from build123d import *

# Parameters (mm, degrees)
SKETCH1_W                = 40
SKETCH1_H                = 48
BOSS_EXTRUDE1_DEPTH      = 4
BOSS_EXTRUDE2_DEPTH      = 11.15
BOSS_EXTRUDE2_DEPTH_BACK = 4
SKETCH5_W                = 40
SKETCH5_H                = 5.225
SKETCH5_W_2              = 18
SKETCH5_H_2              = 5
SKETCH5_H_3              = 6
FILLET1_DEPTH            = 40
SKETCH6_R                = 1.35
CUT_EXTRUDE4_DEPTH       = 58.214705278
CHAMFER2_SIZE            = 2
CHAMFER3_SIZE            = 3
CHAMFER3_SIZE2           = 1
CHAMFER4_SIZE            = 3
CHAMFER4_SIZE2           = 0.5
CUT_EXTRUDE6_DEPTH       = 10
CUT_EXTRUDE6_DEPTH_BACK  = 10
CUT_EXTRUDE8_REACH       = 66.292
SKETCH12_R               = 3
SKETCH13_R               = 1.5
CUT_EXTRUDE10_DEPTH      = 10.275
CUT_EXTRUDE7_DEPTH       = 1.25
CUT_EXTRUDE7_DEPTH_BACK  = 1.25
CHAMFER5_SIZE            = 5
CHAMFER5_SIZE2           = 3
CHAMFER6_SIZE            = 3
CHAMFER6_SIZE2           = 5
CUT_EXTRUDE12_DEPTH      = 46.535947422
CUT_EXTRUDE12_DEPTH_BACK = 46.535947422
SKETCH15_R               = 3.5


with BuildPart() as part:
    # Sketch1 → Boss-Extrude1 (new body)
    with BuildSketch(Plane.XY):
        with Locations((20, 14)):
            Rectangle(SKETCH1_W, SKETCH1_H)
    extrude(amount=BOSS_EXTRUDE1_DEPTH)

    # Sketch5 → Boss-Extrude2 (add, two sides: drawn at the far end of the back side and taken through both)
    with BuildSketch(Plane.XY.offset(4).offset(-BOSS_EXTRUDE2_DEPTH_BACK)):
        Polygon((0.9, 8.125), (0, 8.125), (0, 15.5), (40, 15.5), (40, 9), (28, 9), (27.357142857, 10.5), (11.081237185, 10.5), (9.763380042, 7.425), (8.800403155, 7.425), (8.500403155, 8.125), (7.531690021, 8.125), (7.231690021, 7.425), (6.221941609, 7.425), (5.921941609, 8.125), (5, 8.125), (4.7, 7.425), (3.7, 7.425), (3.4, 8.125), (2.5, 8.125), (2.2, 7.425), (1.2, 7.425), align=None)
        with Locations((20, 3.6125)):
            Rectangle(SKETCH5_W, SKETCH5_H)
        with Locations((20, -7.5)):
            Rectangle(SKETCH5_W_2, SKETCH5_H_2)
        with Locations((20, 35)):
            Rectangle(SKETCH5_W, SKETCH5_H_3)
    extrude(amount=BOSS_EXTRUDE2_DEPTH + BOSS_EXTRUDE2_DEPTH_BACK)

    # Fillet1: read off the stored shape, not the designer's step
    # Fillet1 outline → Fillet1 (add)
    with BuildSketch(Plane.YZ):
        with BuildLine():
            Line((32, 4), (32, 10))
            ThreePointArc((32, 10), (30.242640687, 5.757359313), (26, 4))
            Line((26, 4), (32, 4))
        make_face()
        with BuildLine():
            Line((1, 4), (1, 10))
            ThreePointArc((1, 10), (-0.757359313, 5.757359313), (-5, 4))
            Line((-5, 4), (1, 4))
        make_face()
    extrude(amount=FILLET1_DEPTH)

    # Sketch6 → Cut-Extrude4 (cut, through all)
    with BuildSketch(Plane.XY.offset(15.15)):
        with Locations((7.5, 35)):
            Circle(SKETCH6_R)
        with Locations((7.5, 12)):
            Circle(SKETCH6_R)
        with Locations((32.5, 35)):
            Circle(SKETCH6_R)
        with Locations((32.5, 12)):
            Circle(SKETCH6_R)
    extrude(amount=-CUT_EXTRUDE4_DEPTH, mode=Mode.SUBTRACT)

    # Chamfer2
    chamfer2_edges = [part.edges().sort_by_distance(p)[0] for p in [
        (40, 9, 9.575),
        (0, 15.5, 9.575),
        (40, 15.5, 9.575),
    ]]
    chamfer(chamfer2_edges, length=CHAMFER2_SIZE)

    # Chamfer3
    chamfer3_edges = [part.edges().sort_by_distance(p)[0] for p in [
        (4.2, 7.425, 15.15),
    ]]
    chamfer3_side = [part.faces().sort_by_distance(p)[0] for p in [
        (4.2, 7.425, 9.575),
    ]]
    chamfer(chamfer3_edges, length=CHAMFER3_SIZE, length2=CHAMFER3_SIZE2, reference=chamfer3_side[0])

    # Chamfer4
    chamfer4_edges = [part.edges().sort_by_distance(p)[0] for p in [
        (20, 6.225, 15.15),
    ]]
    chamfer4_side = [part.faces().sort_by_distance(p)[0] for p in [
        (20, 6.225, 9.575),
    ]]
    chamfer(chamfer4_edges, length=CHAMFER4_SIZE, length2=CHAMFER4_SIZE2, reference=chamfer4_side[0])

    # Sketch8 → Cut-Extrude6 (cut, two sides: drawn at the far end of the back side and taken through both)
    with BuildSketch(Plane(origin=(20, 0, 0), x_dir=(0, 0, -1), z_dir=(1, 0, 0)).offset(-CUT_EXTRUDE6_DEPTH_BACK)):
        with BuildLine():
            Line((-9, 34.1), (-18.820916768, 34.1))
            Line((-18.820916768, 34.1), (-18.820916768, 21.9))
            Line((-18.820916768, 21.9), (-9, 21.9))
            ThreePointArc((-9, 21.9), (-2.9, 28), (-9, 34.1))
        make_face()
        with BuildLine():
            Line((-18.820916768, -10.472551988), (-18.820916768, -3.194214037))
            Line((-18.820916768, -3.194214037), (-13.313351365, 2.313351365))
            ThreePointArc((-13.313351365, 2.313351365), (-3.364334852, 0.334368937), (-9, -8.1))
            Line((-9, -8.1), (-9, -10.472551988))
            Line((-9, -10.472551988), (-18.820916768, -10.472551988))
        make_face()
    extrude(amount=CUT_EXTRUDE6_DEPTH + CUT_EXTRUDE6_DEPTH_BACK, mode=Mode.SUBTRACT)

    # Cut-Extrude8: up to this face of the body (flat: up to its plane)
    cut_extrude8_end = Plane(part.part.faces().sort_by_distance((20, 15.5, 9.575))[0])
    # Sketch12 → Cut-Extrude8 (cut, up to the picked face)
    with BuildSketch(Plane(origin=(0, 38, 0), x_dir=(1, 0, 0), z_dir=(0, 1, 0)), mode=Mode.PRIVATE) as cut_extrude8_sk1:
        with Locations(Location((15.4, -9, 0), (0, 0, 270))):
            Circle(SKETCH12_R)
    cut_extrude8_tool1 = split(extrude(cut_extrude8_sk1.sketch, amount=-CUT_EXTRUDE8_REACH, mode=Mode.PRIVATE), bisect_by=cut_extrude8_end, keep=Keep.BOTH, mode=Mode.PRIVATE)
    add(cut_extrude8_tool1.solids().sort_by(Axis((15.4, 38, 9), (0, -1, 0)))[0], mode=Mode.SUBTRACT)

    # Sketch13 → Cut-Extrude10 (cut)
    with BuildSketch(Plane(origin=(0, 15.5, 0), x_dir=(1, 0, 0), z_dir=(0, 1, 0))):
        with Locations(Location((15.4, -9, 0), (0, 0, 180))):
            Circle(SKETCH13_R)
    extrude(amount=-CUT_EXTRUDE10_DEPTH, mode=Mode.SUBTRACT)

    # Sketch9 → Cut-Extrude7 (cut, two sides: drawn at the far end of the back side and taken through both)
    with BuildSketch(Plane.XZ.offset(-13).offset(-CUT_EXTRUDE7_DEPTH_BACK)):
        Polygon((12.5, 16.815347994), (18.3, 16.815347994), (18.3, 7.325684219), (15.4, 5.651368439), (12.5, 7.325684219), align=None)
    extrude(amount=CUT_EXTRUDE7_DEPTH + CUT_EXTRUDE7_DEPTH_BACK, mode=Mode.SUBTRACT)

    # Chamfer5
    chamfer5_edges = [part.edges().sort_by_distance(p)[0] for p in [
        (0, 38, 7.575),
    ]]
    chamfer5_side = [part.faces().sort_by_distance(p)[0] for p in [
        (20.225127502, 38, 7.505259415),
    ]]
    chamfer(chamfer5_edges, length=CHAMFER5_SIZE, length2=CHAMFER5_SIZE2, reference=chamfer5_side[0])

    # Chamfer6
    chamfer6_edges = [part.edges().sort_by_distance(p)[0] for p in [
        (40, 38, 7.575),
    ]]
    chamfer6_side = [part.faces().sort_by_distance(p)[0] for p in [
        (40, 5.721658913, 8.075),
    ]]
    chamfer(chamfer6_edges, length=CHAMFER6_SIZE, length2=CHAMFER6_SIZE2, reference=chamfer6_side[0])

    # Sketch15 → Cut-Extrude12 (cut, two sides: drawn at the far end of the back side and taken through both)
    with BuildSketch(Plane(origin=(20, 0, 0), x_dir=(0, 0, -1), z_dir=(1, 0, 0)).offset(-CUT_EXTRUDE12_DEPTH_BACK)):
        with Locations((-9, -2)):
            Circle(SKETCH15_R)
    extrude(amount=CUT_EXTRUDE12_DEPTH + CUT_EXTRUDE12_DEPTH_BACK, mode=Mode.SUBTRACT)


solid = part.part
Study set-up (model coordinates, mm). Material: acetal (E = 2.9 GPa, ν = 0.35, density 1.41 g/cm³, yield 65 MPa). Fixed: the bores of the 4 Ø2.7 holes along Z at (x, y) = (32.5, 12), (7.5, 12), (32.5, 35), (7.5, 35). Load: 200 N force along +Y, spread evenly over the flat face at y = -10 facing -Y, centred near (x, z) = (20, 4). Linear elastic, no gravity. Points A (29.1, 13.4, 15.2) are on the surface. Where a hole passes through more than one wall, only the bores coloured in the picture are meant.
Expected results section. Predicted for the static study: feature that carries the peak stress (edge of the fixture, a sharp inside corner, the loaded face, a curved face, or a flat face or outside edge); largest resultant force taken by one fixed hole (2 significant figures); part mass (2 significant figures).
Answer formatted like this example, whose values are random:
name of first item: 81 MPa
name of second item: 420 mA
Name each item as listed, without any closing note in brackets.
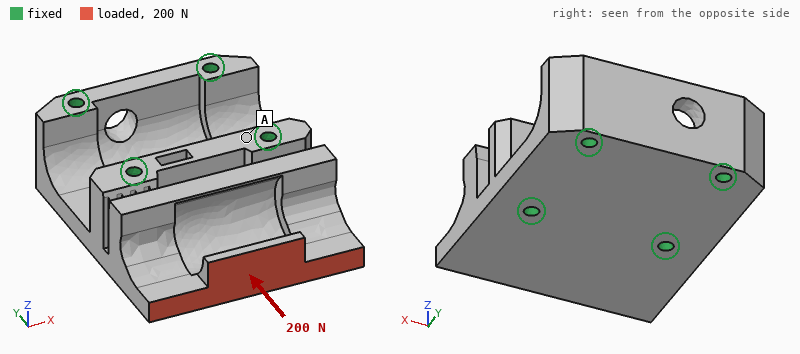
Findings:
feature that carries the peak stress: a curved face
largest resultant force taken by one fixed hole: 89 N
part mass: 20 g
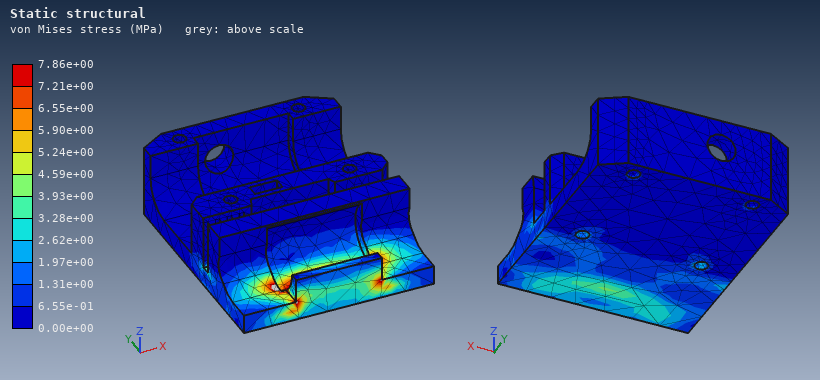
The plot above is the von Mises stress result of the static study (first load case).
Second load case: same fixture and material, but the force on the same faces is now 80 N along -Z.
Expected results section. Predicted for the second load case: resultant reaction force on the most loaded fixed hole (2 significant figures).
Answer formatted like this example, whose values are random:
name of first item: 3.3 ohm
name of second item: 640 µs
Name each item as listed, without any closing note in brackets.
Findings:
resultant reaction force on the most loaded fixed hole: 49 N
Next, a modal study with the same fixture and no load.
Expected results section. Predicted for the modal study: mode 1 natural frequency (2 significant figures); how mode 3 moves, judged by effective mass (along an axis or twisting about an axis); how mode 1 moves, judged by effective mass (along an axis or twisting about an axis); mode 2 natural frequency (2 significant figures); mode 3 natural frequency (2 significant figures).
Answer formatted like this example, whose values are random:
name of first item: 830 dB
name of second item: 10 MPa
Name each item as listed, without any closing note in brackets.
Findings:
mode 1 natural frequency: 1700 Hz
how mode 3 moves, judged by effective mass: along X
how mode 1 moves, judged by effective mass: along Z
mode 2 natural frequency: 3000 Hz
mode 3 natural frequency: 5900 Hz
